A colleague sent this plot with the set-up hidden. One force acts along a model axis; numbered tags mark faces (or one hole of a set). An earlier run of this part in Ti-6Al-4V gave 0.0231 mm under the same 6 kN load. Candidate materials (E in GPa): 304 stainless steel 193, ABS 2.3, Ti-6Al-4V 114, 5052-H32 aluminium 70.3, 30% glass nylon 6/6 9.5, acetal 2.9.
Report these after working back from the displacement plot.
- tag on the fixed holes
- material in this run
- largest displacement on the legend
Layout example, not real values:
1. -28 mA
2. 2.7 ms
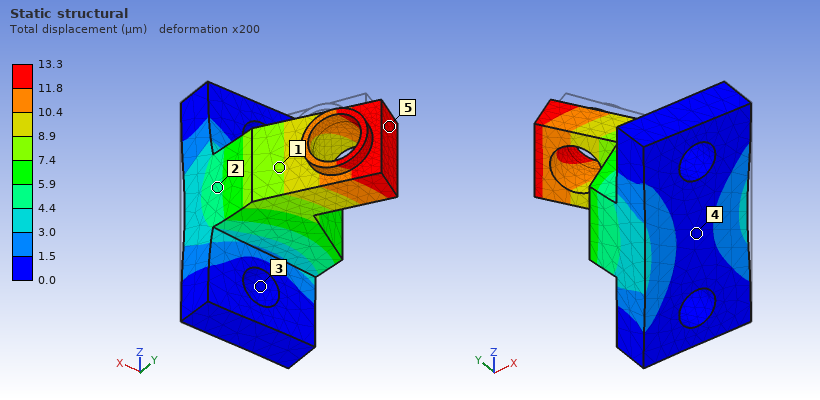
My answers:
1. 3
2. 304 stainless steel
3. 13.3 µm
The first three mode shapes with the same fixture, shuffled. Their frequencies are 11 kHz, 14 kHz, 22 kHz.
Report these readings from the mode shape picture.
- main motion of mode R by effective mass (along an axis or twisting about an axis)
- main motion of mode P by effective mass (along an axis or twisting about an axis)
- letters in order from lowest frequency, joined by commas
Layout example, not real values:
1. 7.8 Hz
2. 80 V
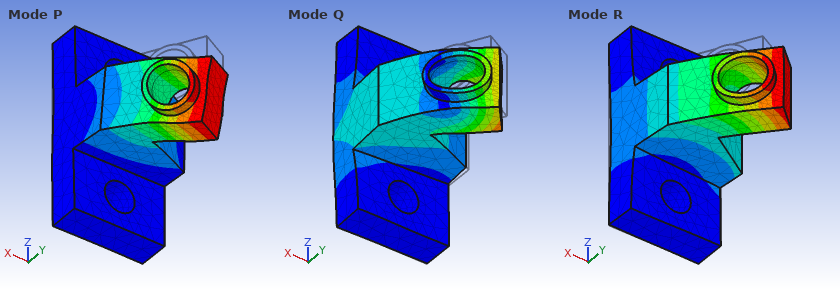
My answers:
1. along X
2. along Z
3. R, P, Q
